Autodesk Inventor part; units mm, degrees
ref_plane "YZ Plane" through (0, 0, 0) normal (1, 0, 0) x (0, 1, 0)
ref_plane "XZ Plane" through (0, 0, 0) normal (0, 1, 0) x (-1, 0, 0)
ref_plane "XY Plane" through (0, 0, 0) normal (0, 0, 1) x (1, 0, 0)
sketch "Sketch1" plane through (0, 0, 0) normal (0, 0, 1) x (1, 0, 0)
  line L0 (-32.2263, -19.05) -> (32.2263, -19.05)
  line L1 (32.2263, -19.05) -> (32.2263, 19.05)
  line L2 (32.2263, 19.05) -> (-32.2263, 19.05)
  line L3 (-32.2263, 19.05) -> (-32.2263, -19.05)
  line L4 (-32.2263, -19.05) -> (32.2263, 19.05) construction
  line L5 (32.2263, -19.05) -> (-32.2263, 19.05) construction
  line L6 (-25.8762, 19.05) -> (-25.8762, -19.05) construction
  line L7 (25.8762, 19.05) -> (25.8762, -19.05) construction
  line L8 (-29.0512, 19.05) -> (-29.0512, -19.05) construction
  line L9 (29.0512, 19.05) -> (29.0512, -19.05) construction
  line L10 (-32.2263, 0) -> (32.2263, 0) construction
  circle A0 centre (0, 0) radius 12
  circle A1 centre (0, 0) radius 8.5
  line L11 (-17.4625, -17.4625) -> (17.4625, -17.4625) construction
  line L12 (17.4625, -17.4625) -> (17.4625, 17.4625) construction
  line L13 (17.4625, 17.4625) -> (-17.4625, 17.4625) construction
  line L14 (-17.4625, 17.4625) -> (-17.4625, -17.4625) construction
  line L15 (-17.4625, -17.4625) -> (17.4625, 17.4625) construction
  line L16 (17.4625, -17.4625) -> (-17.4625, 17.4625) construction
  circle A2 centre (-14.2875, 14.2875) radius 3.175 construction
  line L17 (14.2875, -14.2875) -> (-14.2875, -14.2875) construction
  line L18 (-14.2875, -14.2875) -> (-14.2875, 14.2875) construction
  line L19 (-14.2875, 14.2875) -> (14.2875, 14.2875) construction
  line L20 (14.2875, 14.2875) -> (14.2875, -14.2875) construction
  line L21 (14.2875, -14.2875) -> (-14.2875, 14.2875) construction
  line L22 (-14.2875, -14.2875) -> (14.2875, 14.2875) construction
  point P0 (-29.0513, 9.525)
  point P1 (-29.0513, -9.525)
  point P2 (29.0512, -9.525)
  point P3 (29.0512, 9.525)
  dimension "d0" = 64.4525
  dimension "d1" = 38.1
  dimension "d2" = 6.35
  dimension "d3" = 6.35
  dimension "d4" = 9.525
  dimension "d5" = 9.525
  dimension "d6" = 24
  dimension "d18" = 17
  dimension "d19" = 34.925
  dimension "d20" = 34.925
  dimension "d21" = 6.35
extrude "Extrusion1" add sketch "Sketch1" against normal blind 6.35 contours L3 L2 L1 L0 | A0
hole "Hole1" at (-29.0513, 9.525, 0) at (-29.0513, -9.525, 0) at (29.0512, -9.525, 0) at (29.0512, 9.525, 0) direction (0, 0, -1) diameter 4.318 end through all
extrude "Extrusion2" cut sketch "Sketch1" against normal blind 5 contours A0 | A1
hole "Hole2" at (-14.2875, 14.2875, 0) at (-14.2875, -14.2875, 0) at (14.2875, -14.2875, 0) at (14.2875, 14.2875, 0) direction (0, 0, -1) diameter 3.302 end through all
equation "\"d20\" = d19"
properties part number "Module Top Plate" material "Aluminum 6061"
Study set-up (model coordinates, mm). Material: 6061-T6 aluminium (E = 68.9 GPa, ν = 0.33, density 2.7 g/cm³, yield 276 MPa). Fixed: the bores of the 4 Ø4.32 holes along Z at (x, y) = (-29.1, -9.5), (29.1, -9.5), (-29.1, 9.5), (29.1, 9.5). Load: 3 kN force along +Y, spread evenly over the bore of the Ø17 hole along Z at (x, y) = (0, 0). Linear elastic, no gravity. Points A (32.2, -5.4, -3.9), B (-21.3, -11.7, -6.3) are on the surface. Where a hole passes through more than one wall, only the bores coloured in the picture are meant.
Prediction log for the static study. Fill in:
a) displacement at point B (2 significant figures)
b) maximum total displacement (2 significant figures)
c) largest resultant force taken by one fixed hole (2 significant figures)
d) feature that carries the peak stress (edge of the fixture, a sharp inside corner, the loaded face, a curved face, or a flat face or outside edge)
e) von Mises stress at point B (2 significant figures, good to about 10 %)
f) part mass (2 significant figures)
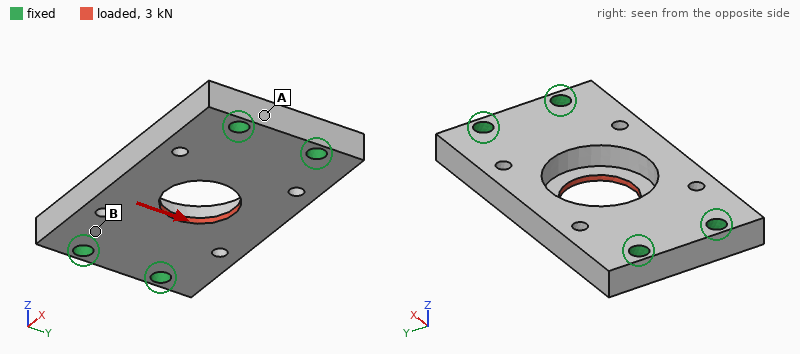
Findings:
4.0 µm
18 µm
990 N
a sharp inside corner
15 MPa
34 g
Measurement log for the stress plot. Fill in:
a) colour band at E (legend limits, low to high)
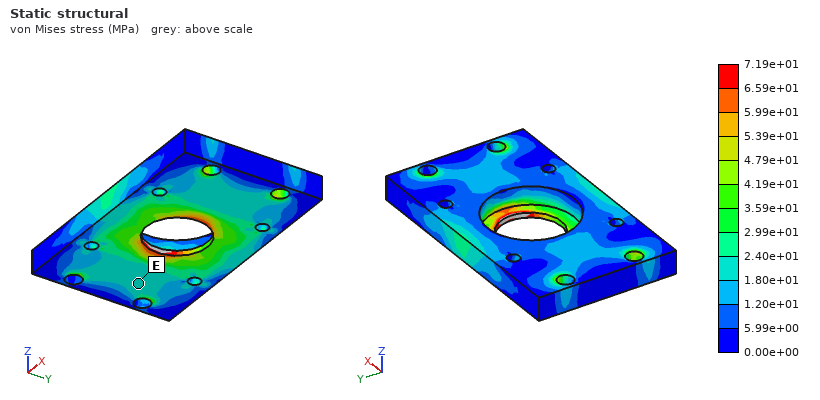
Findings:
1.80e+01 to 2.40e+01 MPa
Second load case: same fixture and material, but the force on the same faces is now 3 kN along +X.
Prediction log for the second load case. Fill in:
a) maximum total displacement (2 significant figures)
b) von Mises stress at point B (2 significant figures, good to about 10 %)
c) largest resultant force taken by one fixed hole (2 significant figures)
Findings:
9.7 µm
12 MPa
760 N
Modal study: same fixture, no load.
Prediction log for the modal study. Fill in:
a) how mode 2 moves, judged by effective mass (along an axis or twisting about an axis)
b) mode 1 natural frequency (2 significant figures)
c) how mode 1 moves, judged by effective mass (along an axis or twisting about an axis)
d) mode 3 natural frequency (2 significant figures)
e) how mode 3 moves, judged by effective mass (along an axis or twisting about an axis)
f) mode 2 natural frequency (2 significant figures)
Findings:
twisting about X
9900 Hz
along Z
20 kHz
twisting about Y
11 kHz
